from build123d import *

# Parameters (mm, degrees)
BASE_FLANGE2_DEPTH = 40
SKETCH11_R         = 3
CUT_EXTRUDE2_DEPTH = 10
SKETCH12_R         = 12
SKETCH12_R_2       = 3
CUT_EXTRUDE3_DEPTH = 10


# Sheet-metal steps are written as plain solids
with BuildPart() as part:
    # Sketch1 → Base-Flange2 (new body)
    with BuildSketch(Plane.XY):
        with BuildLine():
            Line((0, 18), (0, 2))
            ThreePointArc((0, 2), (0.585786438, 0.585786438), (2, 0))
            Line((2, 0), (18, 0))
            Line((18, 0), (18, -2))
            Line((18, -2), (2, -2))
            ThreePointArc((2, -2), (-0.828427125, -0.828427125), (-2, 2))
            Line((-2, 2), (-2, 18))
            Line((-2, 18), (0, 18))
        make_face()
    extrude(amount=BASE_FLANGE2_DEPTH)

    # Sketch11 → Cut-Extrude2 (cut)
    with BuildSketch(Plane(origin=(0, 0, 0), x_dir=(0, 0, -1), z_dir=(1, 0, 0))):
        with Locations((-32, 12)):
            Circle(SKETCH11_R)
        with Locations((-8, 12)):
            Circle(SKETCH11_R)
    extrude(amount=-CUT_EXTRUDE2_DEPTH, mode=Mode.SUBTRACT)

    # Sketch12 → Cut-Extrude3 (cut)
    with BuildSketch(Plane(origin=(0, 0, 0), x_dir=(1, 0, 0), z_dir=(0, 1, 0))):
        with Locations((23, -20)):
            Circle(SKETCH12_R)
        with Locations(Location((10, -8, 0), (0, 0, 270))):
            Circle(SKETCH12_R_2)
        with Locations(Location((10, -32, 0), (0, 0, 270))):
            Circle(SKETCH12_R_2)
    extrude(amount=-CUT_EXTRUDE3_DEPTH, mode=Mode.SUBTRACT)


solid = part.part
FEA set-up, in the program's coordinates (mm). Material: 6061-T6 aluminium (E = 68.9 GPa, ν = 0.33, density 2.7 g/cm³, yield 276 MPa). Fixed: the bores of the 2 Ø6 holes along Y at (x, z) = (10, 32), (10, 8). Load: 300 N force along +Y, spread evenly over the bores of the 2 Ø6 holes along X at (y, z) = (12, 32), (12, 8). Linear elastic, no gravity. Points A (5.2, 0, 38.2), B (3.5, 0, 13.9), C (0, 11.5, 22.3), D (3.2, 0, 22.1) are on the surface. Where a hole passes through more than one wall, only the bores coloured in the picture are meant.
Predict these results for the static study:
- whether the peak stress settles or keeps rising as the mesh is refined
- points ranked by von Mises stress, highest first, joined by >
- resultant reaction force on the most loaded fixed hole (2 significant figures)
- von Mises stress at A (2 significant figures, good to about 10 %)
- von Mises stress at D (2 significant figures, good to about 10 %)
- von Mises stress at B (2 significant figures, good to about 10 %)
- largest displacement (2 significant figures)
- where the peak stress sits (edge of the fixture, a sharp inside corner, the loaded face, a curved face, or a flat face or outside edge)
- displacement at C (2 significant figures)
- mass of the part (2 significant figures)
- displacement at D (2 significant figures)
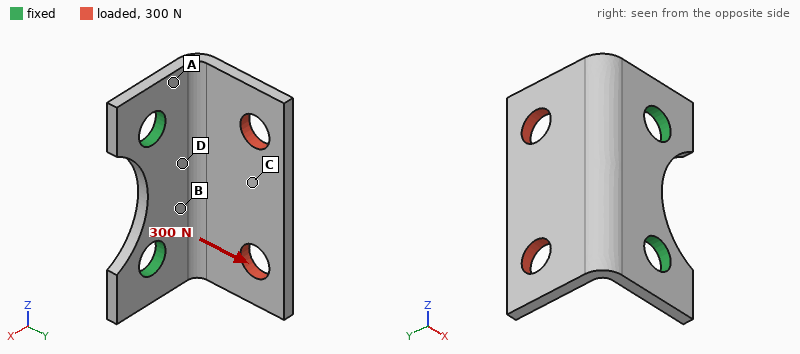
keeps rising
A > B > D > C
150 N
58 MPa
32 MPa
42 MPa
0.14 mm
edge of the fixture
0.094 mm
6.7 g
0.023 mm
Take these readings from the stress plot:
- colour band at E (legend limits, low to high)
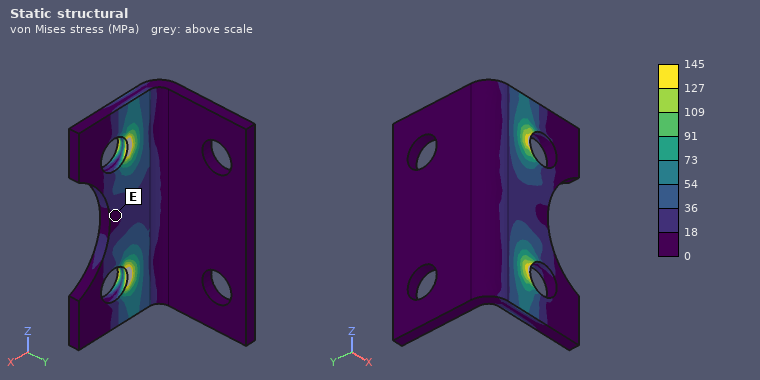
0 to 18 MPa
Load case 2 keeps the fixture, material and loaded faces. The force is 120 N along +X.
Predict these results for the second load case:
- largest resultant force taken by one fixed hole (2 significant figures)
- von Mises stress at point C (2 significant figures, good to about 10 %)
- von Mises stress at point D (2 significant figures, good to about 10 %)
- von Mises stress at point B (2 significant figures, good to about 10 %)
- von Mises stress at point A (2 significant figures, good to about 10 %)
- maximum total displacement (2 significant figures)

62 N
11 MPa
45 MPa
51 MPa
51 MPa
0.21 mm
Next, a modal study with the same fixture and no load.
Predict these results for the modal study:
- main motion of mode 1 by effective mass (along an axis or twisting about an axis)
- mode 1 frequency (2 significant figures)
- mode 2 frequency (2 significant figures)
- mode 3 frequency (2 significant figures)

along X
2800 Hz
4800 Hz
8700 Hz
